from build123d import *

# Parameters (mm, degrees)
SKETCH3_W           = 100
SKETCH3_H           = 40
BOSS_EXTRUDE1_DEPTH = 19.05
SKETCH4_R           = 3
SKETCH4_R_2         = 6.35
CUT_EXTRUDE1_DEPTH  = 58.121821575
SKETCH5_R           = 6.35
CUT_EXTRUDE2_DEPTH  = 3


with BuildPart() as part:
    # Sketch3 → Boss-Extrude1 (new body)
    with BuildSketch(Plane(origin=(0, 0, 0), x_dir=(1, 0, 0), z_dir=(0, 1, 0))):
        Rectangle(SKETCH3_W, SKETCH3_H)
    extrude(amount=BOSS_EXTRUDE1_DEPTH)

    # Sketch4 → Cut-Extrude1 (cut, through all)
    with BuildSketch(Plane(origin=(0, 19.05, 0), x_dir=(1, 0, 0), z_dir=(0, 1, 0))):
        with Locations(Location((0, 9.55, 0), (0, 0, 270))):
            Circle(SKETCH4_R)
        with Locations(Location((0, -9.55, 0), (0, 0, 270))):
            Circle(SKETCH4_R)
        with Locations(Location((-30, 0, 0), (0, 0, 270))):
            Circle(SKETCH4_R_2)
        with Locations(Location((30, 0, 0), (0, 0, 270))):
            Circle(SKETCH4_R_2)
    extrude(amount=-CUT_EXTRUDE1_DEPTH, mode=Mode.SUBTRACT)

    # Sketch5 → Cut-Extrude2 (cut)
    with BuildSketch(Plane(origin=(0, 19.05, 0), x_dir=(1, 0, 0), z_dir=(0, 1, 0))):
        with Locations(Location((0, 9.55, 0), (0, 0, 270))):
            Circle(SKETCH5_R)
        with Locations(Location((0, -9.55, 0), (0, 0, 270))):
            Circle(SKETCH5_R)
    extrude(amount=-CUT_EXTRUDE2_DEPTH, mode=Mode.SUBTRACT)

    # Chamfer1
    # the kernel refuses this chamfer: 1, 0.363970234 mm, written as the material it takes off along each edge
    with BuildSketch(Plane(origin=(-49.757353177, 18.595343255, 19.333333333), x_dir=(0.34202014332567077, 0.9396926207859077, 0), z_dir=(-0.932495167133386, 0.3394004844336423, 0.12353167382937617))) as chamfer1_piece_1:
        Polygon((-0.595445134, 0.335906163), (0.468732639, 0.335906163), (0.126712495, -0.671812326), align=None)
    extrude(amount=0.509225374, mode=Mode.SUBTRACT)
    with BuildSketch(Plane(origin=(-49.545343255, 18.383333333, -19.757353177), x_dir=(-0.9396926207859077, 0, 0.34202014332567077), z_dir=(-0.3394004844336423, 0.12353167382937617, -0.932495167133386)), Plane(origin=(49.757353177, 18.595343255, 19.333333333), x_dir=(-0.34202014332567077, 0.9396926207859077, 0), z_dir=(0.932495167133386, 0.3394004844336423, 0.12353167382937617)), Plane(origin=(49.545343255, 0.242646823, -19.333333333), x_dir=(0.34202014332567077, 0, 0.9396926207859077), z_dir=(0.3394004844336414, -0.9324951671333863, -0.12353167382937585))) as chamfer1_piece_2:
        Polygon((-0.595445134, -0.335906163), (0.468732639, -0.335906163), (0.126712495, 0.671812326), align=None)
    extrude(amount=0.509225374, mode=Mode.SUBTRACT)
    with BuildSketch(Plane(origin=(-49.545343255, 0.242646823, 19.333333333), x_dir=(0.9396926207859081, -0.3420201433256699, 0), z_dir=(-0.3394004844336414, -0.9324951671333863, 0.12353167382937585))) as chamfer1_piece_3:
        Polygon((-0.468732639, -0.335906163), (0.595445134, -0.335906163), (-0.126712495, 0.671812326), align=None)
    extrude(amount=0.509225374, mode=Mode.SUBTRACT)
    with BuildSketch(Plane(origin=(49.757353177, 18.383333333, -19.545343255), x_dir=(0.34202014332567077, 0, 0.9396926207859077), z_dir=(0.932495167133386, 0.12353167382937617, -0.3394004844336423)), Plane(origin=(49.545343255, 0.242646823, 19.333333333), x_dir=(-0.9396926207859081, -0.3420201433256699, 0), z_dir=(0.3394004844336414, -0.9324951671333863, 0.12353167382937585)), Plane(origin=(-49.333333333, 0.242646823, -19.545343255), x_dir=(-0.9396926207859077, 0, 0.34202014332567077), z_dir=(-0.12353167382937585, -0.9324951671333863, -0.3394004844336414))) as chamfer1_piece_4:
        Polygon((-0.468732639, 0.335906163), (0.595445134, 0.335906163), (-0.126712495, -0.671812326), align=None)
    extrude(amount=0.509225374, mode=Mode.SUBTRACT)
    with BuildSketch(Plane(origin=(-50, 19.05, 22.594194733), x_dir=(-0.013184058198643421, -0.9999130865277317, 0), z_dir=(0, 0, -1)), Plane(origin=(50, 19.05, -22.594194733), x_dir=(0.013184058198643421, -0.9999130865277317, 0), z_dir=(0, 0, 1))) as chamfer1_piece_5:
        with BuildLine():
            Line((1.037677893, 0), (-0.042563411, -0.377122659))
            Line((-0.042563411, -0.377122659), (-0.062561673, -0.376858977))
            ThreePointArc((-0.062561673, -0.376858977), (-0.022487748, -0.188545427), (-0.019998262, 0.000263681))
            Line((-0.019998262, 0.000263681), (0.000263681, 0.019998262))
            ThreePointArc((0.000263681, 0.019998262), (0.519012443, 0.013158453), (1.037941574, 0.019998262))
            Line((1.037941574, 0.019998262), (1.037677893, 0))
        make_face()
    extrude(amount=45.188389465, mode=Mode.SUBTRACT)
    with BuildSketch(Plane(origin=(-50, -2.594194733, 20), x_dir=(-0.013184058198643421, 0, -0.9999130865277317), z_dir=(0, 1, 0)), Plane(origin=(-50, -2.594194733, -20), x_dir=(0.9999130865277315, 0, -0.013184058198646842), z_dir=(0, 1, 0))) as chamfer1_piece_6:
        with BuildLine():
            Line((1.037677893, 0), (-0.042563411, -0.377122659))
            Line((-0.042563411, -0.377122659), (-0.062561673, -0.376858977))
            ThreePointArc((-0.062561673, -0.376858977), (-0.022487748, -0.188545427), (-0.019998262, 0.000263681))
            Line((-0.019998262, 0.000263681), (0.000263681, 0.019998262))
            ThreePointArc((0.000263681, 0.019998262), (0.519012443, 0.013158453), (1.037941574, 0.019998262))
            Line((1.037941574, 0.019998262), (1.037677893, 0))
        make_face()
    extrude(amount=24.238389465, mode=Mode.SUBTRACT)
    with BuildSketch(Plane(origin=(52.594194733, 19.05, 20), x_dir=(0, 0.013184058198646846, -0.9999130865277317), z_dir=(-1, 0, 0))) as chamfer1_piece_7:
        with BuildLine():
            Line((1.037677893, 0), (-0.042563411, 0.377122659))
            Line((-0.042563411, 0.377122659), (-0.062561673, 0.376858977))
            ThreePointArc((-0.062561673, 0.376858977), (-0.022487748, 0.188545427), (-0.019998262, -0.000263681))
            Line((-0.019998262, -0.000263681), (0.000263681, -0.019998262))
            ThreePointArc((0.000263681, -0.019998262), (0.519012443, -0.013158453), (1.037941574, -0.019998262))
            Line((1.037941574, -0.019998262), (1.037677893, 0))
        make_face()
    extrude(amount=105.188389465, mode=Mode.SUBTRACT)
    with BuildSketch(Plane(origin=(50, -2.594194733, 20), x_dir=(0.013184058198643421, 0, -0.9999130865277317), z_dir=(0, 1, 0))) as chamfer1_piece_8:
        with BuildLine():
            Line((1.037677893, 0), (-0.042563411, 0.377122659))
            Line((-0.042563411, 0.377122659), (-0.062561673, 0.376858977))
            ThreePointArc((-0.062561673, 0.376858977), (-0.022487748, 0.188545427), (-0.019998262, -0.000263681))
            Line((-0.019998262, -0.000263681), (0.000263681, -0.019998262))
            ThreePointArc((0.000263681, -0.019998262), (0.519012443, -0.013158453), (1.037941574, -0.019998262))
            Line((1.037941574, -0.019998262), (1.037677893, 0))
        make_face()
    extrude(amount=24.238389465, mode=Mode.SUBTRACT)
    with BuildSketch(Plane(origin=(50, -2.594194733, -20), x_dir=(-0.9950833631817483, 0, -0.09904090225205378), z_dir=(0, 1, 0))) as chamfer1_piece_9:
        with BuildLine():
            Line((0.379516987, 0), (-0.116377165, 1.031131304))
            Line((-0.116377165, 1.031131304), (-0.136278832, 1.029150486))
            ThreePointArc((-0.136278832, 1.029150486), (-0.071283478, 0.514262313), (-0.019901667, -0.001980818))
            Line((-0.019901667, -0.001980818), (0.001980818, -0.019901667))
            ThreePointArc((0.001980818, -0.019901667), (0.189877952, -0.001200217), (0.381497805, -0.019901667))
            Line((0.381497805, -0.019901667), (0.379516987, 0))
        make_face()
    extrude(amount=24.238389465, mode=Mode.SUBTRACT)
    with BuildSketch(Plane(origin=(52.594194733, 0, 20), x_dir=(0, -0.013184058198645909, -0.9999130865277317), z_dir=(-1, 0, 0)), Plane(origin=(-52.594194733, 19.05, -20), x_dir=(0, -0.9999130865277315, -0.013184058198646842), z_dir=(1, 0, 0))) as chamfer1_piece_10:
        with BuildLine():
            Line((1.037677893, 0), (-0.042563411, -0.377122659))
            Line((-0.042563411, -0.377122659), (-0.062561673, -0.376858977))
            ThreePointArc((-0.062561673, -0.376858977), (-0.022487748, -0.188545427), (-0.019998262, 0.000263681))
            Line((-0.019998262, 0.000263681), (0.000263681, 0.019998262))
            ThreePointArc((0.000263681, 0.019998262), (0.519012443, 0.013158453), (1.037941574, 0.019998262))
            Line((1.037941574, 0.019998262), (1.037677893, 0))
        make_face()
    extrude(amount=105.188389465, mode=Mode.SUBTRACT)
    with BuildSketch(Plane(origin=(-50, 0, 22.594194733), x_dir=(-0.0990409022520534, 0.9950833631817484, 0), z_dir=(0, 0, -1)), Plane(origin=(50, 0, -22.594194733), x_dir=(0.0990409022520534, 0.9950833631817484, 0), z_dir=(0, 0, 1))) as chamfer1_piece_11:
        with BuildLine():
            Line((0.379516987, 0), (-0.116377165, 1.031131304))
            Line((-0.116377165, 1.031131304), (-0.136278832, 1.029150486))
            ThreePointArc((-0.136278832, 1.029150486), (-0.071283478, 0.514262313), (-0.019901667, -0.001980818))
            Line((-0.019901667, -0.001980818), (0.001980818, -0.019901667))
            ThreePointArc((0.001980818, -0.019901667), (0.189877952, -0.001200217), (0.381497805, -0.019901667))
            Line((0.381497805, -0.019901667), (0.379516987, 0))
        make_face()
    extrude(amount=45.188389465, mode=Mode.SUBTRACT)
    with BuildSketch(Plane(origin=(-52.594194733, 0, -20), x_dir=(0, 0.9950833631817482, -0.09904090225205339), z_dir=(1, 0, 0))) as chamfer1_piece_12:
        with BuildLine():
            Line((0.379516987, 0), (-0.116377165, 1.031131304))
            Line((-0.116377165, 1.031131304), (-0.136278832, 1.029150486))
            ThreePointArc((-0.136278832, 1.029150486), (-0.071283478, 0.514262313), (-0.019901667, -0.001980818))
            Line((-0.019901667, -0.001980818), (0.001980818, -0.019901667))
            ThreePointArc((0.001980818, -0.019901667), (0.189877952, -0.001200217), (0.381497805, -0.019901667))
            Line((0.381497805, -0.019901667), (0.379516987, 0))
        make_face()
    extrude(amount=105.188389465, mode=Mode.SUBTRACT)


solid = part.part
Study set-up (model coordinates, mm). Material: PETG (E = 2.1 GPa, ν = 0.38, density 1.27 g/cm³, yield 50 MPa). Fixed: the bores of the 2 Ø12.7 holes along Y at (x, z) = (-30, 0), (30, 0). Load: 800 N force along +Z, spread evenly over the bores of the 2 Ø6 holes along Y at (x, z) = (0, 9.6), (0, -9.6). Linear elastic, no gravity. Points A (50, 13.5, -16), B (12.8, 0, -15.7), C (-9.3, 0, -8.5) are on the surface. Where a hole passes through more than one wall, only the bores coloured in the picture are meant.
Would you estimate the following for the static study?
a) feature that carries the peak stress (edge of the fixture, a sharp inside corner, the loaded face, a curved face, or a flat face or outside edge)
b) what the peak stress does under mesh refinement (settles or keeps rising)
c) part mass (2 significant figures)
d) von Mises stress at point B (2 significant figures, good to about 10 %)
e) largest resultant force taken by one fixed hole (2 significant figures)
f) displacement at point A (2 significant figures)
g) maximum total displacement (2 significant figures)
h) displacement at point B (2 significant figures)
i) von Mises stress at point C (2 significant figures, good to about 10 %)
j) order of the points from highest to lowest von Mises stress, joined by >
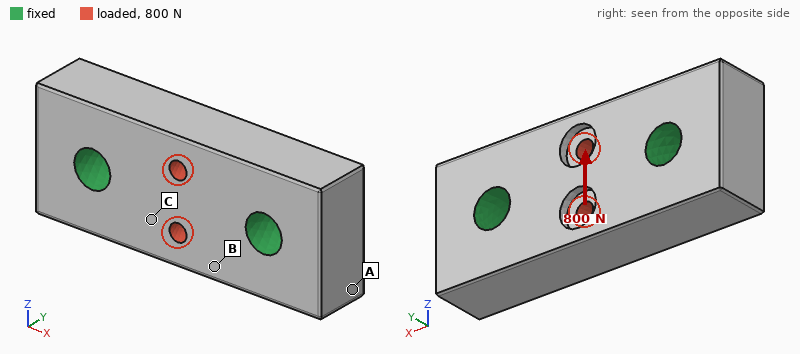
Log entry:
edge of the fixture
keeps rising
88 g
1.00 MPa
400 N
7.8 µm
33 µm
19 µm
1.2 MPa
C > B > A
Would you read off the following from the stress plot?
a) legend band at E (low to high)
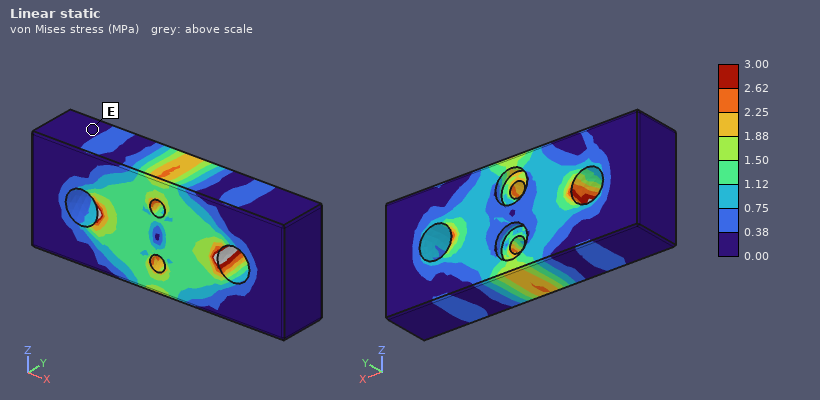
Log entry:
0.00 to 0.38 MPa
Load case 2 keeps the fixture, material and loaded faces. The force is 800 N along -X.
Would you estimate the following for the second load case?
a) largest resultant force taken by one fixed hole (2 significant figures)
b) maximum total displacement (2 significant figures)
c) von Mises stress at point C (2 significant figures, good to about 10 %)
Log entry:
400 N
11 µm
0.99 MPa
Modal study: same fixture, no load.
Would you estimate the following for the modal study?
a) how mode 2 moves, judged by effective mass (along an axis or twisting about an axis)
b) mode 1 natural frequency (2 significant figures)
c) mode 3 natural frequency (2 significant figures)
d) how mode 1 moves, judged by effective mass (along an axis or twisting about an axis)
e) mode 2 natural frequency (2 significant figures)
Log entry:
twisting about X
4800 Hz
5300 Hz
along Y
5100 Hz
